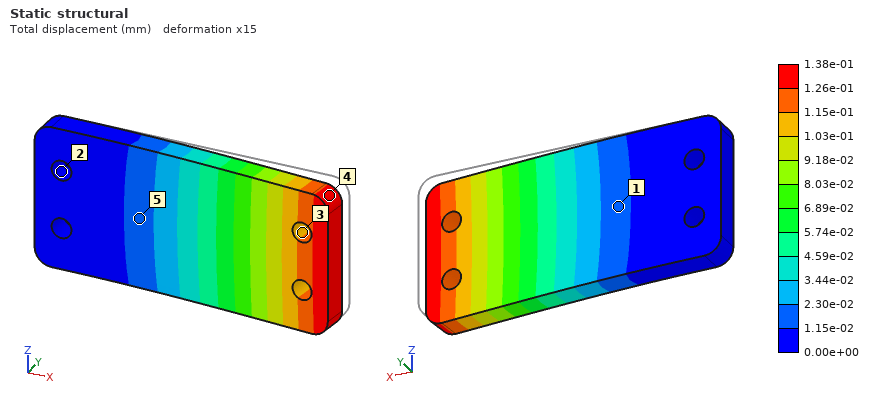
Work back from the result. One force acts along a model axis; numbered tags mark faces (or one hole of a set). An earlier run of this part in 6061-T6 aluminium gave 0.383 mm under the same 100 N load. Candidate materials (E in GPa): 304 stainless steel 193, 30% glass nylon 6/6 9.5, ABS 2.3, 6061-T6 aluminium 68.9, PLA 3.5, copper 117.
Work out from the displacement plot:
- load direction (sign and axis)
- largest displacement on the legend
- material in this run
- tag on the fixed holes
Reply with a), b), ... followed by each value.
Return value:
a) -Y
b) 1.38e-01 mm
c) 304 stainless steel
d) 2
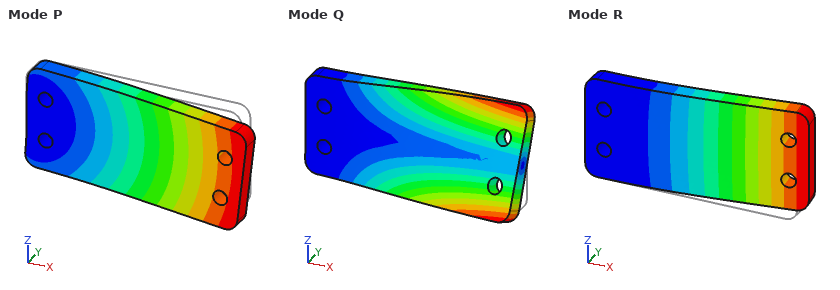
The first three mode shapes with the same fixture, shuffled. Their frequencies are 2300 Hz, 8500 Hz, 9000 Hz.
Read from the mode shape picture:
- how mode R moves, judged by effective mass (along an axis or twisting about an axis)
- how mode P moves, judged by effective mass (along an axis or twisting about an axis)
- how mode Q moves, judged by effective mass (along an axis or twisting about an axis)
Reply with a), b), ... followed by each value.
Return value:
a) along Y
b) along Z
c) twisting about X
